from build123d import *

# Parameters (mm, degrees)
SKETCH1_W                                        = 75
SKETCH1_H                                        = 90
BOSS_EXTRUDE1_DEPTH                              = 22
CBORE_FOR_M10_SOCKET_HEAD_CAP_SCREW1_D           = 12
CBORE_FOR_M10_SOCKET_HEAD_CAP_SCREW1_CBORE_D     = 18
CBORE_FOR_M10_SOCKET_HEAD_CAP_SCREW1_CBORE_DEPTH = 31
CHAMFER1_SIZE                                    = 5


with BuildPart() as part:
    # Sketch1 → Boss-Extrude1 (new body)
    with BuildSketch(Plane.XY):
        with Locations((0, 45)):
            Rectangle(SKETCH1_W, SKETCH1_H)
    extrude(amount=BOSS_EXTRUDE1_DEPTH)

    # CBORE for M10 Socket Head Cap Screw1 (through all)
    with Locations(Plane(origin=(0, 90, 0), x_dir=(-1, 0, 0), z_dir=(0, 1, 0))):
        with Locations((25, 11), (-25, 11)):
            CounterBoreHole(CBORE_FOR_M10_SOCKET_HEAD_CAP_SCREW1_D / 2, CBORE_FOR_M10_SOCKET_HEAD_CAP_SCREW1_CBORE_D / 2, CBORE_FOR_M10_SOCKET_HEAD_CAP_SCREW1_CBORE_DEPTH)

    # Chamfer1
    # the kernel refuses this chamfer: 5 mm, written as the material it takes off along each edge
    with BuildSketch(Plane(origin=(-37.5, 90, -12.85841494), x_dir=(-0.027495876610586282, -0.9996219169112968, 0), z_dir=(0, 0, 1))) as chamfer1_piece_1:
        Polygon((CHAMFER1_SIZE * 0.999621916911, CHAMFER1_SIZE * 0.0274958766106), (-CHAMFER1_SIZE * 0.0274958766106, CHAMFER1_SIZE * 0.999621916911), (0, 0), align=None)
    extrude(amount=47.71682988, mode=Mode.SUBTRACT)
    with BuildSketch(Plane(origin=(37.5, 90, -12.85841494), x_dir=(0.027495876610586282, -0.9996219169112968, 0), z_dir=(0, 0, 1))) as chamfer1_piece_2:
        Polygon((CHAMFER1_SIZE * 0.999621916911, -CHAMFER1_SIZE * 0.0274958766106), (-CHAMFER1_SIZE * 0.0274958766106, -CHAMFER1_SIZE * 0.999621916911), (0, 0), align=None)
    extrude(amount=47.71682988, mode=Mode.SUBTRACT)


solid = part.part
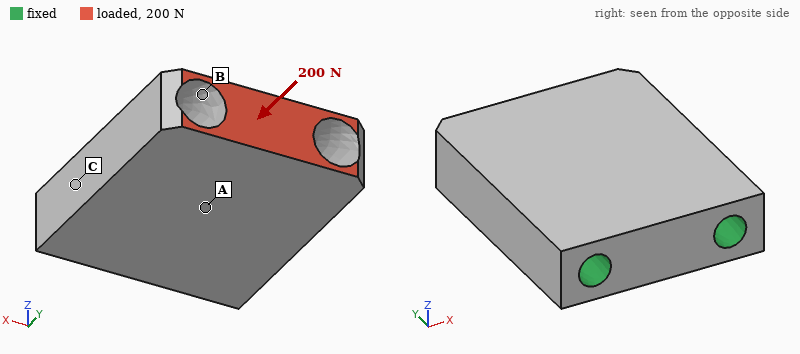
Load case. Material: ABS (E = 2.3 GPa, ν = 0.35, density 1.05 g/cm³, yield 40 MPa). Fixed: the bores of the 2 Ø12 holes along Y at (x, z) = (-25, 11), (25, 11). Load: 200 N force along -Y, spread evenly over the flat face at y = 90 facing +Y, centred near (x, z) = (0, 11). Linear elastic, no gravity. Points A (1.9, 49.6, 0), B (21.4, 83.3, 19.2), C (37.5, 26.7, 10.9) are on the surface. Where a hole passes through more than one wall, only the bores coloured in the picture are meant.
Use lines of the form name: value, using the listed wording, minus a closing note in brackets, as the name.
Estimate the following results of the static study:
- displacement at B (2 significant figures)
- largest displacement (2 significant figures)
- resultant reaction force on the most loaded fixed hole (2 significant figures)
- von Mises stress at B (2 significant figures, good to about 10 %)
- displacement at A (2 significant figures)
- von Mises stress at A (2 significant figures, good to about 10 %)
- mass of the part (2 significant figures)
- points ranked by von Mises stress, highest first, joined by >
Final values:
displacement at B: 3.2 µm
largest displacement: 4.2 µm
resultant reaction force on the most loaded fixed hole: 110 N
von Mises stress at B: 0.23 MPa
displacement at A: 1.3 µm
von Mises stress at A: 0.11 MPa
mass of the part: 120 g
points ranked by von Mises stress, highest first, joined by >: B > A > C
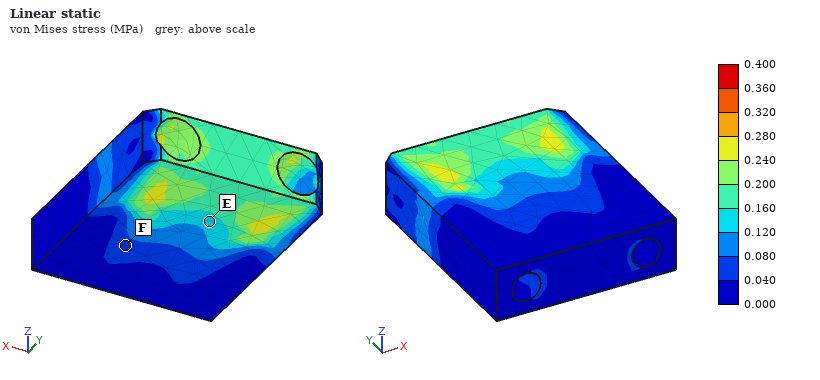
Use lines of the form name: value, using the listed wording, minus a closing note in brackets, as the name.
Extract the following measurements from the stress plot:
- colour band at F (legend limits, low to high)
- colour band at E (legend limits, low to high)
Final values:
colour band at F: 0.040 to 0.080 MPa
colour band at E: 0.120 to 0.160 MPa
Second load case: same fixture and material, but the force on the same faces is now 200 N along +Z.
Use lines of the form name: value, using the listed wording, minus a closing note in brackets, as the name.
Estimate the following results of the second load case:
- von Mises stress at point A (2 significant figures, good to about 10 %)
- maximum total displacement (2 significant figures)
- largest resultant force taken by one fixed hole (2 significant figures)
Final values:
von Mises stress at point A: 0.98 MPa
maximum total displacement: 67 µm
largest resultant force taken by one fixed hole: 100 N
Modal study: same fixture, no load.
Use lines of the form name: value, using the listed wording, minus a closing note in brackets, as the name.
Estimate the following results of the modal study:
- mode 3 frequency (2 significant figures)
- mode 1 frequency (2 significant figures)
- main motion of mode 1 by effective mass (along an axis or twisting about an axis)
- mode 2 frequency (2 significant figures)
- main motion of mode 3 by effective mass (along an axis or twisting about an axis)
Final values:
mode 3 frequency: 4700 Hz
mode 1 frequency: 2500 Hz
main motion of mode 1 by effective mass: along Z
mode 2 frequency: 4200 Hz
main motion of mode 3 by effective mass: along X
